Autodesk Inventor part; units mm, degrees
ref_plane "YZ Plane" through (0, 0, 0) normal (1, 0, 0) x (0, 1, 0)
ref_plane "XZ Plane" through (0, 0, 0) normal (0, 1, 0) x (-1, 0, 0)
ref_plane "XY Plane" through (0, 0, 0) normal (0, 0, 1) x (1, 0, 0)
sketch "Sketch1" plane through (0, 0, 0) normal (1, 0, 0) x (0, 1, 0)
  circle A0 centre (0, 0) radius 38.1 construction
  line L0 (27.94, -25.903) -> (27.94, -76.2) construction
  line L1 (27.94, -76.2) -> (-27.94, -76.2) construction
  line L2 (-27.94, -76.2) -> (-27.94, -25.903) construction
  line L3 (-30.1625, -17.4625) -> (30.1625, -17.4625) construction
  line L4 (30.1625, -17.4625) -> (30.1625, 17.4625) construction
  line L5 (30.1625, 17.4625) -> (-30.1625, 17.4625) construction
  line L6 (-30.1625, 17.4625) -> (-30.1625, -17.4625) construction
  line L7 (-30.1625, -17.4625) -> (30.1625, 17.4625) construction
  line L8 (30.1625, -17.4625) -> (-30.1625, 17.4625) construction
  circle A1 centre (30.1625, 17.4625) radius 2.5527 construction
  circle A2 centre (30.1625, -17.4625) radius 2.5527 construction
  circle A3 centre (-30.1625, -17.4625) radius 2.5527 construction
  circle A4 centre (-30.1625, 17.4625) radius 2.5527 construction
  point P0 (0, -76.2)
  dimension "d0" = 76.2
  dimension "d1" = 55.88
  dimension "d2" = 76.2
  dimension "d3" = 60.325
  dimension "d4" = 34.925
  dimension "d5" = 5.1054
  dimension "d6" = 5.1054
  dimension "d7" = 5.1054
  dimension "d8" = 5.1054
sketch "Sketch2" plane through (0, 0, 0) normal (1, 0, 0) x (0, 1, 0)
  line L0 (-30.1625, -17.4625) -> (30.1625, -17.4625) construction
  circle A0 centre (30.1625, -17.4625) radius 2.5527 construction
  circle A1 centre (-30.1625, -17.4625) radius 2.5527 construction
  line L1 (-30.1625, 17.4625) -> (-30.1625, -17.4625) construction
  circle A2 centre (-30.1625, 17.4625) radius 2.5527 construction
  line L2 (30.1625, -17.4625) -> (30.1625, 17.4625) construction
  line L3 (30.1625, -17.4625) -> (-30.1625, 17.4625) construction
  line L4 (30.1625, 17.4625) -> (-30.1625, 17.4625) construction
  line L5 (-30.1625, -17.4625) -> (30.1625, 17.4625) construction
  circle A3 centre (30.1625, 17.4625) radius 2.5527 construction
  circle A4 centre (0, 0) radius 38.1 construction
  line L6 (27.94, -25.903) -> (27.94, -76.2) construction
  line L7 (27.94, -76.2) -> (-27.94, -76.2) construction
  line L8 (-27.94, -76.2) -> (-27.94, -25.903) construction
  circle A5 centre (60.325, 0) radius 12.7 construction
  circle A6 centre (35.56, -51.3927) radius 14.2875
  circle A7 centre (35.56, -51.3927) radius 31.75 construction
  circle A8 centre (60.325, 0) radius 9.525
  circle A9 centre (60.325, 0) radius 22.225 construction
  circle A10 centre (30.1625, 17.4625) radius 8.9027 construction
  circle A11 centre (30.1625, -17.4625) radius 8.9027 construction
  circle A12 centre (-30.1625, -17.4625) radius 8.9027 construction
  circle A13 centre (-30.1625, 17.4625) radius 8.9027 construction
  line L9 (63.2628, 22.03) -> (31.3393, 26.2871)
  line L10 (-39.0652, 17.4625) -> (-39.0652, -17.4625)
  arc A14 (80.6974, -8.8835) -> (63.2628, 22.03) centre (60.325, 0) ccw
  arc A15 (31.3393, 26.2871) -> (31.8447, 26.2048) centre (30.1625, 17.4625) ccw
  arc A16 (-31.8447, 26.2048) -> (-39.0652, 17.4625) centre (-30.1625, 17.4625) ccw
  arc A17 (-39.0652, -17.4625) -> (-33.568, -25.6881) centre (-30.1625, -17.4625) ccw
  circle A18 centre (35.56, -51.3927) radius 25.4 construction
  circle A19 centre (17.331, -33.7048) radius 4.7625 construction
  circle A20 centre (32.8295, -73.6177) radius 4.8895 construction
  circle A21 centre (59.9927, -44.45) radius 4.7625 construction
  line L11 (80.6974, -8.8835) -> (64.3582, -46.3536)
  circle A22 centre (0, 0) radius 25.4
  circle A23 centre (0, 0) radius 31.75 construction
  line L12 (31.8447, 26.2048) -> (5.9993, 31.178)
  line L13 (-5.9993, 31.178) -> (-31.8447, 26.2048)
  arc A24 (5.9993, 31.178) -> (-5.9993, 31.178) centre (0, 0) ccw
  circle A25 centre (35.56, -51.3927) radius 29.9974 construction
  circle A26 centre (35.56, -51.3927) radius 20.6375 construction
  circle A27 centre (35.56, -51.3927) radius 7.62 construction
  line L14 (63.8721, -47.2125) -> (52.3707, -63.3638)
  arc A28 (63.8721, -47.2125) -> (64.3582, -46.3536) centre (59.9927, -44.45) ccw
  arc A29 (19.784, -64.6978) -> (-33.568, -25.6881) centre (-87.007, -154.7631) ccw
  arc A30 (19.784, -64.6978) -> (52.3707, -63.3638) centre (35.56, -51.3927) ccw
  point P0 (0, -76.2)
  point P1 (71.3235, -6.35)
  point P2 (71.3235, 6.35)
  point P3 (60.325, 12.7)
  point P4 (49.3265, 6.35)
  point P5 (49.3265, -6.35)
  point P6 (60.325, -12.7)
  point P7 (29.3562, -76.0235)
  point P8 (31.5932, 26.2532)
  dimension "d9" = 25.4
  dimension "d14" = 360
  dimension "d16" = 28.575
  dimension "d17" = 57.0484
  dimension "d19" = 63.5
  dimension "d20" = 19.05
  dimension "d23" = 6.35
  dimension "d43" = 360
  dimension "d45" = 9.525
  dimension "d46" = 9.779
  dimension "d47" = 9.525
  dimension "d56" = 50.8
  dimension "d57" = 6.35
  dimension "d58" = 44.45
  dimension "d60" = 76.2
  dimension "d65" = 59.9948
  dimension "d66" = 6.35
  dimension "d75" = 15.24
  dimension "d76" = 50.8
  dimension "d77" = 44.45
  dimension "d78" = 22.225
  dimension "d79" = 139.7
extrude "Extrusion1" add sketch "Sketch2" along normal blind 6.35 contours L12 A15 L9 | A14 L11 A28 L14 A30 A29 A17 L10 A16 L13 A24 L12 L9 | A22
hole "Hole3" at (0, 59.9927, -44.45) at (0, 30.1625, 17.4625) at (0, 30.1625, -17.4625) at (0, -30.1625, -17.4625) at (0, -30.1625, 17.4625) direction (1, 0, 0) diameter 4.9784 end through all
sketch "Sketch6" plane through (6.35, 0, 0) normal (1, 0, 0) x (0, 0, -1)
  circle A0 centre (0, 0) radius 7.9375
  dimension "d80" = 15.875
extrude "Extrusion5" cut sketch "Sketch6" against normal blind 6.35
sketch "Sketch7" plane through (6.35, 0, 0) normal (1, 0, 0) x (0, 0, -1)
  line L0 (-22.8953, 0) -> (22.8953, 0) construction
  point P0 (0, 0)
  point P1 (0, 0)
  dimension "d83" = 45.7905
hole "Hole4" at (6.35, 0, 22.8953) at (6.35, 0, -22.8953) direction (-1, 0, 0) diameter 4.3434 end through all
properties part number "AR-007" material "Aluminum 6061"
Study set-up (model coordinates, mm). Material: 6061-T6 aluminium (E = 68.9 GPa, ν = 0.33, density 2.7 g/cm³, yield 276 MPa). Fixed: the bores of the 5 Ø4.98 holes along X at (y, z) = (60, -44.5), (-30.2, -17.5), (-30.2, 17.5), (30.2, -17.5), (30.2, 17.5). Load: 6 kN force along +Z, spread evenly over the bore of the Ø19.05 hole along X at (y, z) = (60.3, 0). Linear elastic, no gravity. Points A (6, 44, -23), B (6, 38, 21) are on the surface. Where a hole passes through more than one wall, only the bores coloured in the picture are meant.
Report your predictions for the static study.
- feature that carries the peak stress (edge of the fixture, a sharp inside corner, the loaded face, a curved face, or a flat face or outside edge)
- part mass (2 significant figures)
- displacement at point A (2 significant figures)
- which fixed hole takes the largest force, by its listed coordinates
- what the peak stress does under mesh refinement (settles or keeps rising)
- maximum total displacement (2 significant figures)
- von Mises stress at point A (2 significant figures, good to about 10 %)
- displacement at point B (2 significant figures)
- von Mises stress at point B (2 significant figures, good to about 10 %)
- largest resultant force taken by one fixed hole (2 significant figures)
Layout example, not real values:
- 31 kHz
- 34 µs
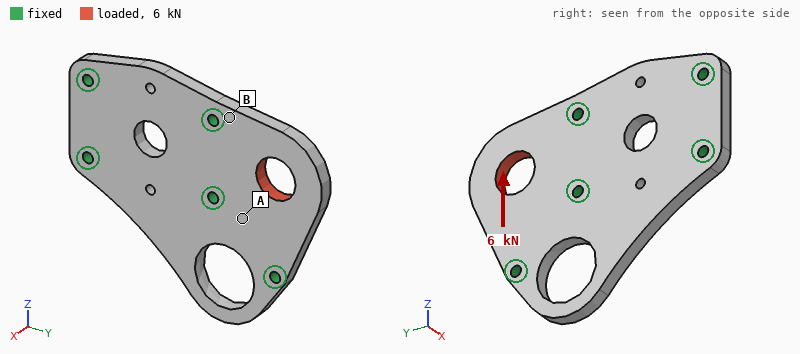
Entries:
- edge of the fixture
- 130 g
- 4.6 µm
- (60, -44.5)
- keeps rising
- 26 µm
- 6.2 MPa
- 5.0 µm
- 19 MPa
- 3.1 kN
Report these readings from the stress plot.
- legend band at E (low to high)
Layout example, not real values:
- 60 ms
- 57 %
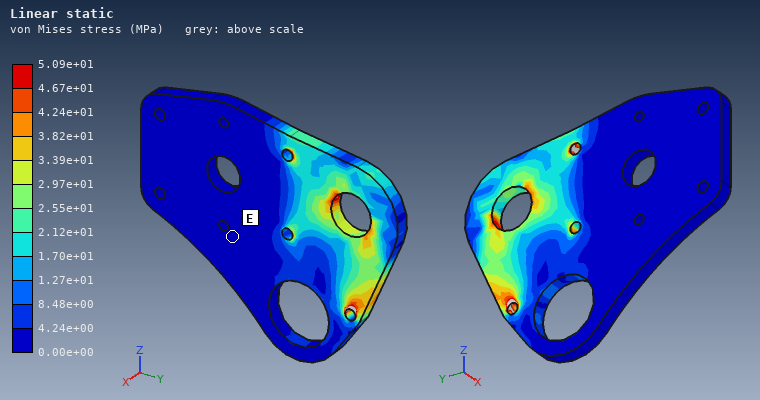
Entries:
- 0.00e+00 to 4.24e+00 MPa
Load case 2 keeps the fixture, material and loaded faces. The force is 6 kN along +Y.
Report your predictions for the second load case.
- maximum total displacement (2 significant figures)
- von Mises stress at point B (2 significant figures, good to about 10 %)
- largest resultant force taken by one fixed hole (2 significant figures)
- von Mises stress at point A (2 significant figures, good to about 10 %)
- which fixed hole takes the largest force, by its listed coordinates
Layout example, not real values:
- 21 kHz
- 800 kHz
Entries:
- 19 µm
- 24 MPa
- 3.0 kN
- 13 MPa
- (30.2, 17.5)
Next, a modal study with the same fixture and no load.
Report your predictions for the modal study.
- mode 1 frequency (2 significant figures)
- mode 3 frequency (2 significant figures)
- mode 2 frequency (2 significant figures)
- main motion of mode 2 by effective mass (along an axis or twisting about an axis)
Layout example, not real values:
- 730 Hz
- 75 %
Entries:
- 3100 Hz
- 6600 Hz
- 3600 Hz
- along X
